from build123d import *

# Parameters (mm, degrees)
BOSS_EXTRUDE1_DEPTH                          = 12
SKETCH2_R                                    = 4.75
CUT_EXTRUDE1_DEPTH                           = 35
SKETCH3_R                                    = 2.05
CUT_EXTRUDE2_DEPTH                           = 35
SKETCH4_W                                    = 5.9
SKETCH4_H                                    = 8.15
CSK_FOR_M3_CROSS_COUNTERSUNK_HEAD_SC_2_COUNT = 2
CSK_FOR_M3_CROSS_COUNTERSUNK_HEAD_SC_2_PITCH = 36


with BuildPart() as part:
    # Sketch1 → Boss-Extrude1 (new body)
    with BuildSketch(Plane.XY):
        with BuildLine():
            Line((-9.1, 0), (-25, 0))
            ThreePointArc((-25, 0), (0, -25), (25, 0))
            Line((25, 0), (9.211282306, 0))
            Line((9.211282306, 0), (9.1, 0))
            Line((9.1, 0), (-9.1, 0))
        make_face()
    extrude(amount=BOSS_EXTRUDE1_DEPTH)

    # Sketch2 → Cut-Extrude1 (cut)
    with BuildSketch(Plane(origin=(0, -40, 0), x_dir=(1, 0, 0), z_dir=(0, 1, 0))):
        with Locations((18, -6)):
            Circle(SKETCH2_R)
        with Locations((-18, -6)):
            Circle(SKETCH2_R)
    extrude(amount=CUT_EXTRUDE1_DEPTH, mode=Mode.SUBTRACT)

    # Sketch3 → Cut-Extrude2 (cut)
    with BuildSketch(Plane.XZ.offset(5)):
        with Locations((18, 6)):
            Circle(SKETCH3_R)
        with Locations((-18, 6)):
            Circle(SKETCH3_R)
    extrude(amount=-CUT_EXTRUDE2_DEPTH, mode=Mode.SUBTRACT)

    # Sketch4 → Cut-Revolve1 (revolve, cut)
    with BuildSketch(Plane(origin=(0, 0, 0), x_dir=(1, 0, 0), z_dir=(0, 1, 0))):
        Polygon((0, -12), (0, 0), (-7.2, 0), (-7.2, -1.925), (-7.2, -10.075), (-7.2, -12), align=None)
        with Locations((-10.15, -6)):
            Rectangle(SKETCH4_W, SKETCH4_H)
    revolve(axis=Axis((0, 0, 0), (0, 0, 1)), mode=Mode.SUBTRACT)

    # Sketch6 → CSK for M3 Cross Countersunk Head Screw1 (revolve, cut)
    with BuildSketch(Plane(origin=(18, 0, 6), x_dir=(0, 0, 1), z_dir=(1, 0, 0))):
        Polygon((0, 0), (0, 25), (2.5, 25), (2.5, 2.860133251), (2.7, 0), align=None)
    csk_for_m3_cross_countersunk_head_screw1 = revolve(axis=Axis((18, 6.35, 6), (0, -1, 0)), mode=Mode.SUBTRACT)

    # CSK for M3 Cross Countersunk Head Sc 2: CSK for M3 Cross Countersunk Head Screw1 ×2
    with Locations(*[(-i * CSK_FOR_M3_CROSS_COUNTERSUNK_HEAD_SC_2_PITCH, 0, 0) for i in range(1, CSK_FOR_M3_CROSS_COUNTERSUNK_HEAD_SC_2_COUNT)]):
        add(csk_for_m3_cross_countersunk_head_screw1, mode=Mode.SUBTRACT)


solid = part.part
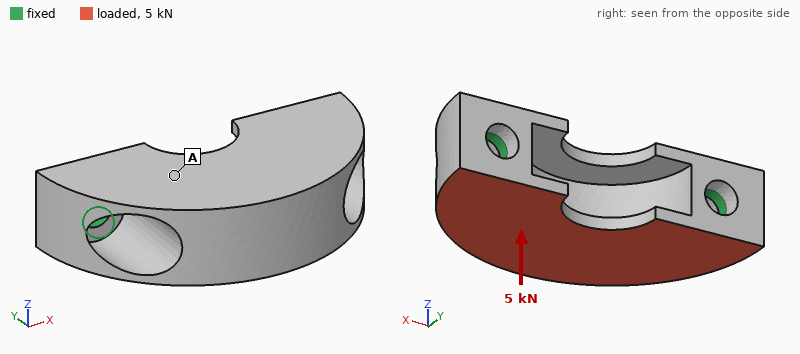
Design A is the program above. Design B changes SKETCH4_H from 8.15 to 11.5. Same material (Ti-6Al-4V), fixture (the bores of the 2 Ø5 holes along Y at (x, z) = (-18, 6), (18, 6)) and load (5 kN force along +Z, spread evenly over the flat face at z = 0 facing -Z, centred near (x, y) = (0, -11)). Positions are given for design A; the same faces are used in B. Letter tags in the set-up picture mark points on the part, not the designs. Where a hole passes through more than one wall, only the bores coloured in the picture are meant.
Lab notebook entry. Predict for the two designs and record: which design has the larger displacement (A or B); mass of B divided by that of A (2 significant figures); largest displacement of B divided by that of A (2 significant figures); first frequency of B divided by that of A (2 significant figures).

B
0.91
17
1.0
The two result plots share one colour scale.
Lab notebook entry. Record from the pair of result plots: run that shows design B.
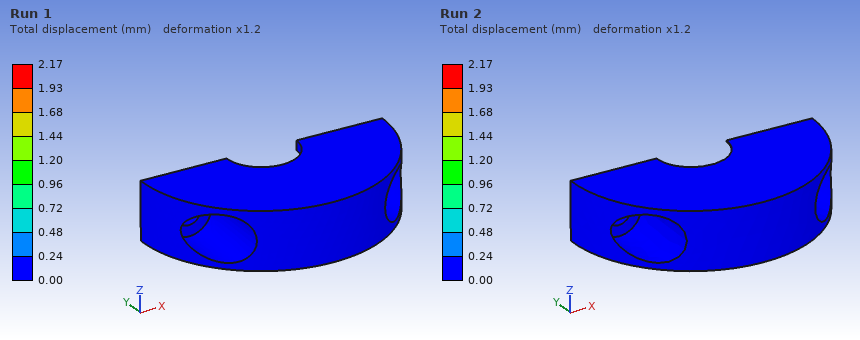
Run 2
